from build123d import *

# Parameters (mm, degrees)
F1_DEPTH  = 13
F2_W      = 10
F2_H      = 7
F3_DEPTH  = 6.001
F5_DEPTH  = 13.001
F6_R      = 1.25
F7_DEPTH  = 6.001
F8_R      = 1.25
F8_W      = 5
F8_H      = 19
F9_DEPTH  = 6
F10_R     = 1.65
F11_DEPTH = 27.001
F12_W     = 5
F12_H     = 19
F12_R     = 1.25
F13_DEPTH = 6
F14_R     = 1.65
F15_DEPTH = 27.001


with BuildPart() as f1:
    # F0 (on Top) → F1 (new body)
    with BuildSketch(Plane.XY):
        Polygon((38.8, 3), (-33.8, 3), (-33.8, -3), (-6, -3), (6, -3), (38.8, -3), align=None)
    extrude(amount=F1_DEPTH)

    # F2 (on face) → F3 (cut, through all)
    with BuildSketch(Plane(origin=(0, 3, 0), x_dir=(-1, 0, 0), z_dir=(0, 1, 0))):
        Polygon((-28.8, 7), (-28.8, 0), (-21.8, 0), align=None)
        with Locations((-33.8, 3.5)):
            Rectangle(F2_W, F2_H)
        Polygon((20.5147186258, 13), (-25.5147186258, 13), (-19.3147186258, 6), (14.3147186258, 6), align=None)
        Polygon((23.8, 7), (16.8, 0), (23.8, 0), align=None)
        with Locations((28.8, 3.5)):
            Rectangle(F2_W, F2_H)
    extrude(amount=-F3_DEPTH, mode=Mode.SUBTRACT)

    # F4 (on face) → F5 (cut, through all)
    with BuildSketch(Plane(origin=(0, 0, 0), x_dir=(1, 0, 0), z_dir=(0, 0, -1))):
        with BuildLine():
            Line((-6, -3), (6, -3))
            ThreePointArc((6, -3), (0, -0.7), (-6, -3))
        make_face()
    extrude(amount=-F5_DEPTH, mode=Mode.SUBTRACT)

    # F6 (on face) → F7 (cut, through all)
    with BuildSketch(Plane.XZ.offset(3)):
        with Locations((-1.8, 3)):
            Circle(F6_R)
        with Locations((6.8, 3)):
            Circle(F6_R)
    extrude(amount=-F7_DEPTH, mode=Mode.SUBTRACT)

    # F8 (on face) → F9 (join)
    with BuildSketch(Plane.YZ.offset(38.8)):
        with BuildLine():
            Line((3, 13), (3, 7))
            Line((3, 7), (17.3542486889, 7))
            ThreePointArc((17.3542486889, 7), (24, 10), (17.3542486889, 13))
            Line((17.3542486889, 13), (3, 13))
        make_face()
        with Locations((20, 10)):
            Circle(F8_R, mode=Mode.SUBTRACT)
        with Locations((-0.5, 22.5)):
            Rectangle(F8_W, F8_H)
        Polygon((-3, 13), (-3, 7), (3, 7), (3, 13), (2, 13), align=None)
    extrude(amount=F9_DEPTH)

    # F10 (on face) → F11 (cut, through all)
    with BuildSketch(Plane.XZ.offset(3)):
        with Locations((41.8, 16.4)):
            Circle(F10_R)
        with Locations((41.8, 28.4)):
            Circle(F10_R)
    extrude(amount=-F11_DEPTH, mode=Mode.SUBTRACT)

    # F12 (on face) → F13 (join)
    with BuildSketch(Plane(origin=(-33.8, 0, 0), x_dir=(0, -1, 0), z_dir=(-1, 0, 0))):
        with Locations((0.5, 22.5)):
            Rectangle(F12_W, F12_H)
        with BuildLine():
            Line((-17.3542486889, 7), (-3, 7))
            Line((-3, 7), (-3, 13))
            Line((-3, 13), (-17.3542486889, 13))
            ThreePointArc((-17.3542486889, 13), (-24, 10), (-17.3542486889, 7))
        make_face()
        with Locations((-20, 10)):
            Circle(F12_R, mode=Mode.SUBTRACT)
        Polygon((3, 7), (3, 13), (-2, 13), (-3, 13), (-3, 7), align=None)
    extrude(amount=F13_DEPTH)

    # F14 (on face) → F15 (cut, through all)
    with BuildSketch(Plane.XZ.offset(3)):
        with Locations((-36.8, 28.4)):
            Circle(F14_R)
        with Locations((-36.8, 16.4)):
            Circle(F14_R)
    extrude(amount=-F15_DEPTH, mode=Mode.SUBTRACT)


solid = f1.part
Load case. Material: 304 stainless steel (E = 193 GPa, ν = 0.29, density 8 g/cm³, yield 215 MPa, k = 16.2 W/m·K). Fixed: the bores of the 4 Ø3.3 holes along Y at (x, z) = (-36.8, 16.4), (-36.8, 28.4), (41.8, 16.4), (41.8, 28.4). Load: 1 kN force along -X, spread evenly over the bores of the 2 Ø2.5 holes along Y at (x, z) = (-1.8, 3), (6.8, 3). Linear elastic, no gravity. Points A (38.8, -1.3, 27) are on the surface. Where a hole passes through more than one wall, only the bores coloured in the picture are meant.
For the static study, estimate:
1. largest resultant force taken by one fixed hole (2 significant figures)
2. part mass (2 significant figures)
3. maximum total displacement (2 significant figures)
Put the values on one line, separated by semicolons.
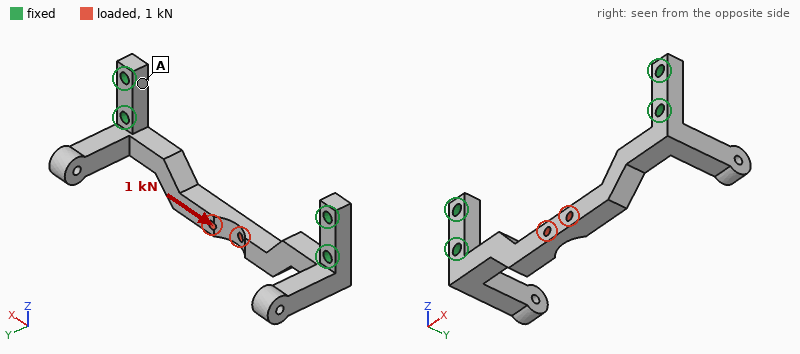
540 N; 45 g; 12 µm
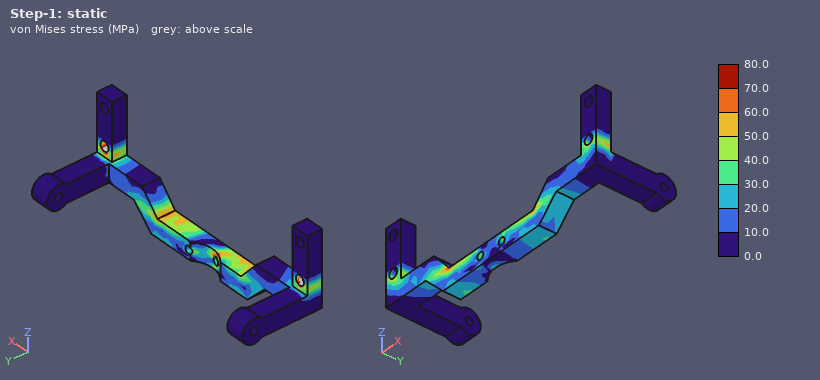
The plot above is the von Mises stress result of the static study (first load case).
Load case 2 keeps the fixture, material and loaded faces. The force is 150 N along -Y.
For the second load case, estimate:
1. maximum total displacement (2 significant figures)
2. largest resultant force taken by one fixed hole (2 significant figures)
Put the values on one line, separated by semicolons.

50 µm; 82 N
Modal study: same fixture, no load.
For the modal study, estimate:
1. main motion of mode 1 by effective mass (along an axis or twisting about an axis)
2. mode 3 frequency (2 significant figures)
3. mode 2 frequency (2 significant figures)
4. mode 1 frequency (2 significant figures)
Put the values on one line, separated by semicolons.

along Y; 5500 Hz; 5400 Hz; 2900 Hz
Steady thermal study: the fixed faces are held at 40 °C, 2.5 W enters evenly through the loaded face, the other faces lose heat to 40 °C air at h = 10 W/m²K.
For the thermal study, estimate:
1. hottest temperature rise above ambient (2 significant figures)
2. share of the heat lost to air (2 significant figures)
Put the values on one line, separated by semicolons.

74 K; 32 %
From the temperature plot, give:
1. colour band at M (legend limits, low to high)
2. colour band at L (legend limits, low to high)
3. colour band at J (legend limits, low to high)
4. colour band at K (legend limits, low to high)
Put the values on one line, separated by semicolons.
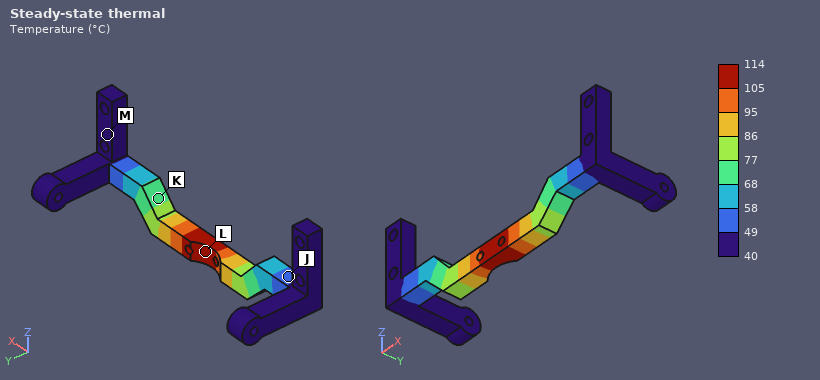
40 to 49 °C; 105 to 114 °C; 49 to 58 °C; 68 to 77 °C
